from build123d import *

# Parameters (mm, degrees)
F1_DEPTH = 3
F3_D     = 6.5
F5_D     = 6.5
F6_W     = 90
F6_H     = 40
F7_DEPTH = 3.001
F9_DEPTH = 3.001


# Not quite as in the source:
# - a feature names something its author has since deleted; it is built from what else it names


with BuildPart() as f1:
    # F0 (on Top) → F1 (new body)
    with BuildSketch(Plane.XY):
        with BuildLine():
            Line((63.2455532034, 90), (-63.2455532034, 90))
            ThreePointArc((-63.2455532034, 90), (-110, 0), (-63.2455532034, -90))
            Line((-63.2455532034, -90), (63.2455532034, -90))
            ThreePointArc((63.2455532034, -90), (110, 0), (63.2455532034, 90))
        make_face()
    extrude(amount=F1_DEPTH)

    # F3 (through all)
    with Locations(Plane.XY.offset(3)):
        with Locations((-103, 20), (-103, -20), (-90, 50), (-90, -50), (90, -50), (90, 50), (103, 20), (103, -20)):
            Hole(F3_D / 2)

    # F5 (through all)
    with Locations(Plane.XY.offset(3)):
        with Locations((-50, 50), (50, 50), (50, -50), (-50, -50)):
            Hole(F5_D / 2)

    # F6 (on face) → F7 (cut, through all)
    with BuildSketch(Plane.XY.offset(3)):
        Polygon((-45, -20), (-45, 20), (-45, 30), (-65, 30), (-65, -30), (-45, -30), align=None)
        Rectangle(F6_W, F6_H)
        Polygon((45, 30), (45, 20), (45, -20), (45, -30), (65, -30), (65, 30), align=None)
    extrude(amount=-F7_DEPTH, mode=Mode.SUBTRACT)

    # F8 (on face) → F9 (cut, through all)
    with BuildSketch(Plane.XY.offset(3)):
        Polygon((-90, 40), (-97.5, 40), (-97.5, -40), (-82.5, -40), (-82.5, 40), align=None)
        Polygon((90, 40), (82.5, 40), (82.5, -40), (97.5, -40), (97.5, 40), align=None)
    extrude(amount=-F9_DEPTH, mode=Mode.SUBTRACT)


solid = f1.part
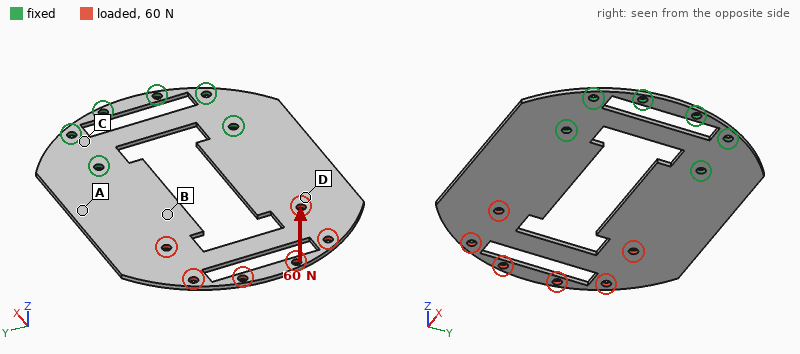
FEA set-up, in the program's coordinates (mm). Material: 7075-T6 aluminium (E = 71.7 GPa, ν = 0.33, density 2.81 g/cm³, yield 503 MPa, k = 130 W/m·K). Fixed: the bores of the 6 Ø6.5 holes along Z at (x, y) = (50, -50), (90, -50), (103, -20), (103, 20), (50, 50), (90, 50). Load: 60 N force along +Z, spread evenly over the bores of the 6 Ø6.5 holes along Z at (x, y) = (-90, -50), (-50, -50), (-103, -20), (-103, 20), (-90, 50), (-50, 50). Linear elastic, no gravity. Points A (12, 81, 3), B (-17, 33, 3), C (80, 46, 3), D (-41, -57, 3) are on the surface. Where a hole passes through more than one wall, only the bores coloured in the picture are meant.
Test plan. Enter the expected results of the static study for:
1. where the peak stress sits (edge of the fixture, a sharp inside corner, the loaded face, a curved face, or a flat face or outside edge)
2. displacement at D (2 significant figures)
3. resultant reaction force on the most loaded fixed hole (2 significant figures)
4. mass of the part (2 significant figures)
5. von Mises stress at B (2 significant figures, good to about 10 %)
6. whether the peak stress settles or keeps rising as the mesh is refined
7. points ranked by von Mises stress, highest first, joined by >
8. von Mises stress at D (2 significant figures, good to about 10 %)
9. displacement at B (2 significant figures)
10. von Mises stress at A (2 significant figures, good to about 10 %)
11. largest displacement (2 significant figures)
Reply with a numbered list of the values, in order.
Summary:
1. edge of the fixture
2. 1.2 mm
3. 59 N
4. 220 g
5. 18 MPa
6. keeps rising
7. A > B > D > C
8. 13 MPa
9. 0.73 mm
10. 26 MPa
11. 3.0 mm
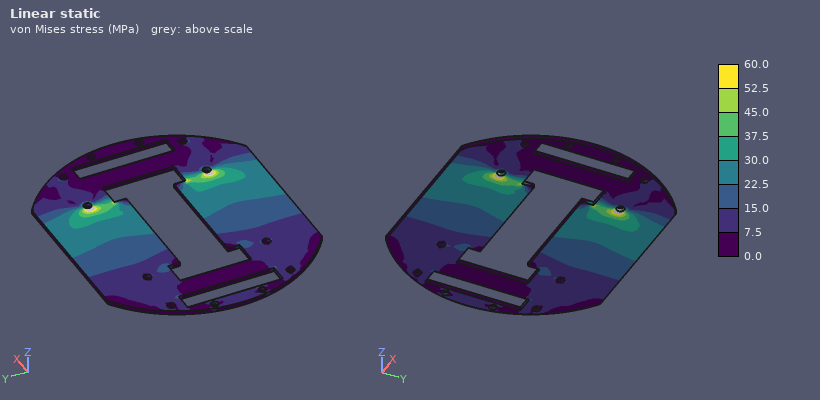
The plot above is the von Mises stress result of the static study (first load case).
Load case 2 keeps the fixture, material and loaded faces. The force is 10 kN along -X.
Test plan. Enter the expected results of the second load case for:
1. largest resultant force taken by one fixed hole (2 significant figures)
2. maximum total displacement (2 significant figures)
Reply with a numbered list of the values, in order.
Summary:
1. 3.9 kN
2. 0.72 mm
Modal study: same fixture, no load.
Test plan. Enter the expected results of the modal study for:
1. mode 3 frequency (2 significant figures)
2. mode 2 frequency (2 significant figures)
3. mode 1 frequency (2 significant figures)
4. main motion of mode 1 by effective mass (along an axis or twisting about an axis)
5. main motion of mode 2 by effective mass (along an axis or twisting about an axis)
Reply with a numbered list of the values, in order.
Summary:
1. 520 Hz
2. 220 Hz
3. 110 Hz
4. along Z
5. twisting about X
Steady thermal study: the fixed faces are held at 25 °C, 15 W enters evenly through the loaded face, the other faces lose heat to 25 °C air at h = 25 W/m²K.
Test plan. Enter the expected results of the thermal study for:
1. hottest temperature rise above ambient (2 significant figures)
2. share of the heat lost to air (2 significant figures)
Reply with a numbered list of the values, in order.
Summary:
1. 42 K
2. 71 %
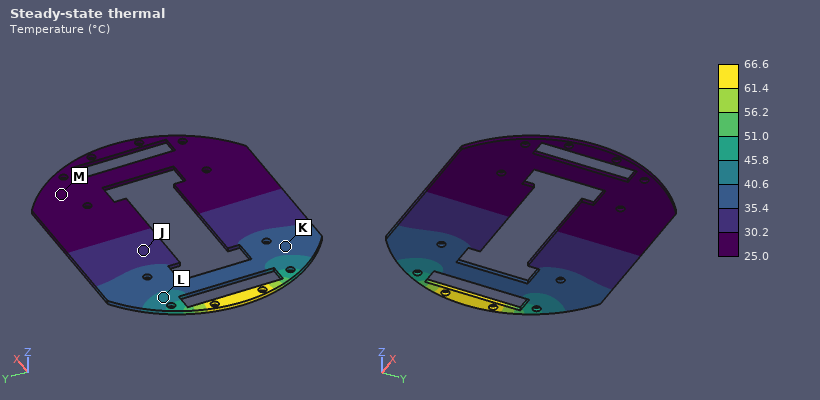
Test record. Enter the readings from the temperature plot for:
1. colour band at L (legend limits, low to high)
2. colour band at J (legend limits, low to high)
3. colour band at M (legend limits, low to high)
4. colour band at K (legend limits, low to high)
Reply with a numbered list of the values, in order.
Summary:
1. 40.6 to 45.8 °C
2. 30.2 to 35.4 °C
3. 25.0 to 30.2 °C
4. 35.4 to 40.6 °C
